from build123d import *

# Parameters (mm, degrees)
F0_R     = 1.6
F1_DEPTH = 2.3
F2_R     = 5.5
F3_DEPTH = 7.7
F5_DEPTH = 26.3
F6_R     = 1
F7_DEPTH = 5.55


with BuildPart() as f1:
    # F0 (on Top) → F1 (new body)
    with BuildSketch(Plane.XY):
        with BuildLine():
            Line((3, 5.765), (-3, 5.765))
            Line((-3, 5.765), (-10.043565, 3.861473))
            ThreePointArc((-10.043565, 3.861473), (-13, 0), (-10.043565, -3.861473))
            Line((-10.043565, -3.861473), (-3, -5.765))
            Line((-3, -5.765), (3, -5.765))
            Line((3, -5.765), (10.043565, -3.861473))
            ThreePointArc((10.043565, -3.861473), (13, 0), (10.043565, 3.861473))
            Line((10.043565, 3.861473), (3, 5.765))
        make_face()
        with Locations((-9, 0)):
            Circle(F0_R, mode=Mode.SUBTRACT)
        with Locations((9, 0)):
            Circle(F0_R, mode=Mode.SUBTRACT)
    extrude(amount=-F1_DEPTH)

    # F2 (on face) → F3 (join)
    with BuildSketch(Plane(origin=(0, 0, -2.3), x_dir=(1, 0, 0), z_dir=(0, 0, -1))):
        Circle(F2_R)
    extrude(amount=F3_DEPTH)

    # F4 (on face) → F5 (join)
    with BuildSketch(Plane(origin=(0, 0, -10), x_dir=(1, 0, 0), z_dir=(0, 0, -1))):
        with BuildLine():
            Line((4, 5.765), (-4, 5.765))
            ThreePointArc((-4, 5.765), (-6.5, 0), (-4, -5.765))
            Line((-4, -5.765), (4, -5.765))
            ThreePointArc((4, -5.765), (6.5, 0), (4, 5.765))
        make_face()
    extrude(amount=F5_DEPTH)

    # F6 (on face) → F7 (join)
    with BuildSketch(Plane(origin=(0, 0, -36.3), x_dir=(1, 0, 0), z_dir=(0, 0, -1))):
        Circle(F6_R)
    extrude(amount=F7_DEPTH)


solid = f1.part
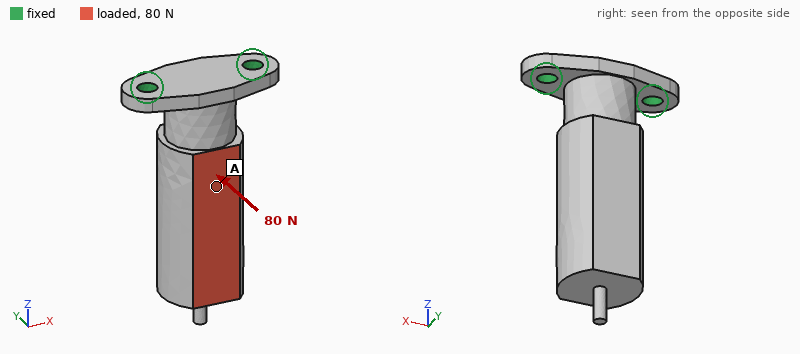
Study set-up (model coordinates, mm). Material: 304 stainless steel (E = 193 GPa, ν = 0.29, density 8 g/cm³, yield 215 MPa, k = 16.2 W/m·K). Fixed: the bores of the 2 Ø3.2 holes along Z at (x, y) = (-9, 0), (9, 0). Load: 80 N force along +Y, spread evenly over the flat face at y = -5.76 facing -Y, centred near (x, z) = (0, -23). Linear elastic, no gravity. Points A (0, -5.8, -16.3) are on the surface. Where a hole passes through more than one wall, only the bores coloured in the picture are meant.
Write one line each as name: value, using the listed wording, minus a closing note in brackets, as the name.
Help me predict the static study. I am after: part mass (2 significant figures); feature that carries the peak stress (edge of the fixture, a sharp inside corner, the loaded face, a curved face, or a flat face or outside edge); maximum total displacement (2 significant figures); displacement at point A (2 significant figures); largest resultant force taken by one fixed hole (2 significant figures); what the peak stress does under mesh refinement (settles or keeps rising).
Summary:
part mass: 38 g
feature that carries the peak stress: edge of the fixture
maximum total displacement: 44 µm
displacement at point A: 17 µm
largest resultant force taken by one fixed hole: 40 N
what the peak stress does under mesh refinement: keeps rising
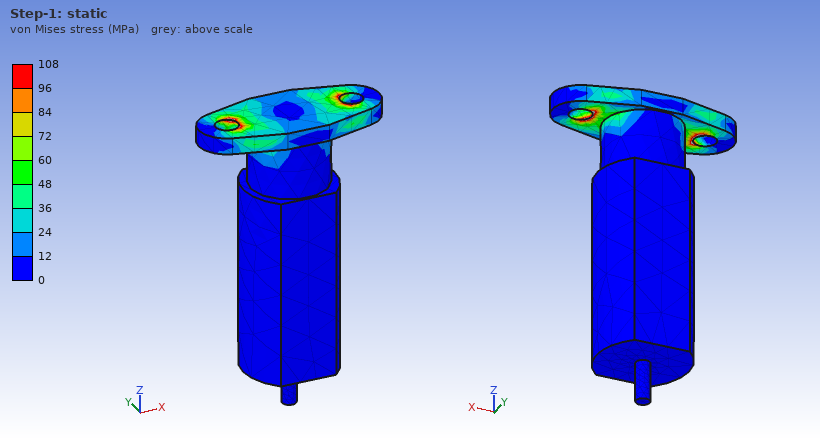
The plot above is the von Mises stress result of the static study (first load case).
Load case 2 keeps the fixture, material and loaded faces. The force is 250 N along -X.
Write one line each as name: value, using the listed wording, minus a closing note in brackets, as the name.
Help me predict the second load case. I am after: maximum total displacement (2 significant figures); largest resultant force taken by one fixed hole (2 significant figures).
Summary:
maximum total displacement: 27 µm
largest resultant force taken by one fixed hole: 440 N
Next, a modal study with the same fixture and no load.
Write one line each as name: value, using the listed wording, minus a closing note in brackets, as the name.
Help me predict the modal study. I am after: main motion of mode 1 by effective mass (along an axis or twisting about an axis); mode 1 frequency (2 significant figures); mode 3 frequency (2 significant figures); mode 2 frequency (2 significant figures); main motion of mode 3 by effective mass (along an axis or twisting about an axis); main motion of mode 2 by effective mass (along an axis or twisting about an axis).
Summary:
main motion of mode 1 by effective mass: along Y
mode 1 frequency: 1600 Hz
mode 3 frequency: 13 kHz
mode 2 frequency: 3700 Hz
main motion of mode 3 by effective mass: along Z
main motion of mode 2 by effective mass: along X
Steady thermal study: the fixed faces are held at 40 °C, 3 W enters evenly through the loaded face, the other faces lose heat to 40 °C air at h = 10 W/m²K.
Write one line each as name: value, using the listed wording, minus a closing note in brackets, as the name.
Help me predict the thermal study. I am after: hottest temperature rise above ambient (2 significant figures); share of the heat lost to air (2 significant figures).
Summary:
hottest temperature rise above ambient: 48 K
share of the heat lost to air: 18 %
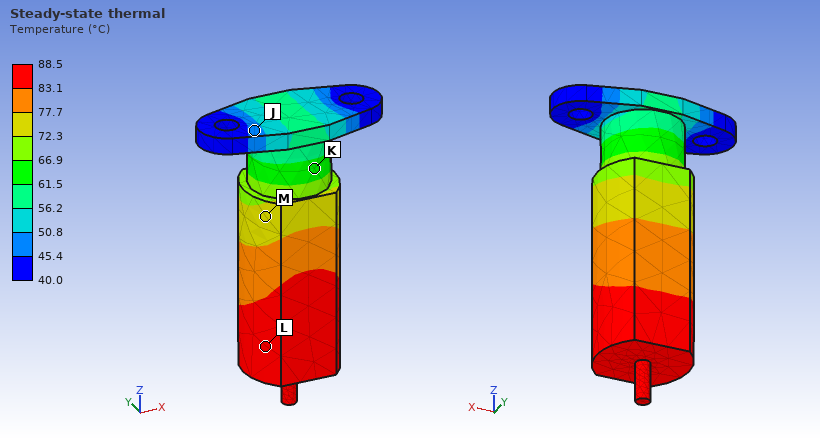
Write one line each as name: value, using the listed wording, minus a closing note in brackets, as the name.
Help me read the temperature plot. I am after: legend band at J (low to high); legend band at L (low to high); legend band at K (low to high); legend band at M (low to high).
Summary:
legend band at J: 45.4 to 50.8 °C
legend band at L: 83.1 to 88.5 °C
legend band at K: 61.5 to 66.9 °C
legend band at M: 72.3 to 77.7 °C
